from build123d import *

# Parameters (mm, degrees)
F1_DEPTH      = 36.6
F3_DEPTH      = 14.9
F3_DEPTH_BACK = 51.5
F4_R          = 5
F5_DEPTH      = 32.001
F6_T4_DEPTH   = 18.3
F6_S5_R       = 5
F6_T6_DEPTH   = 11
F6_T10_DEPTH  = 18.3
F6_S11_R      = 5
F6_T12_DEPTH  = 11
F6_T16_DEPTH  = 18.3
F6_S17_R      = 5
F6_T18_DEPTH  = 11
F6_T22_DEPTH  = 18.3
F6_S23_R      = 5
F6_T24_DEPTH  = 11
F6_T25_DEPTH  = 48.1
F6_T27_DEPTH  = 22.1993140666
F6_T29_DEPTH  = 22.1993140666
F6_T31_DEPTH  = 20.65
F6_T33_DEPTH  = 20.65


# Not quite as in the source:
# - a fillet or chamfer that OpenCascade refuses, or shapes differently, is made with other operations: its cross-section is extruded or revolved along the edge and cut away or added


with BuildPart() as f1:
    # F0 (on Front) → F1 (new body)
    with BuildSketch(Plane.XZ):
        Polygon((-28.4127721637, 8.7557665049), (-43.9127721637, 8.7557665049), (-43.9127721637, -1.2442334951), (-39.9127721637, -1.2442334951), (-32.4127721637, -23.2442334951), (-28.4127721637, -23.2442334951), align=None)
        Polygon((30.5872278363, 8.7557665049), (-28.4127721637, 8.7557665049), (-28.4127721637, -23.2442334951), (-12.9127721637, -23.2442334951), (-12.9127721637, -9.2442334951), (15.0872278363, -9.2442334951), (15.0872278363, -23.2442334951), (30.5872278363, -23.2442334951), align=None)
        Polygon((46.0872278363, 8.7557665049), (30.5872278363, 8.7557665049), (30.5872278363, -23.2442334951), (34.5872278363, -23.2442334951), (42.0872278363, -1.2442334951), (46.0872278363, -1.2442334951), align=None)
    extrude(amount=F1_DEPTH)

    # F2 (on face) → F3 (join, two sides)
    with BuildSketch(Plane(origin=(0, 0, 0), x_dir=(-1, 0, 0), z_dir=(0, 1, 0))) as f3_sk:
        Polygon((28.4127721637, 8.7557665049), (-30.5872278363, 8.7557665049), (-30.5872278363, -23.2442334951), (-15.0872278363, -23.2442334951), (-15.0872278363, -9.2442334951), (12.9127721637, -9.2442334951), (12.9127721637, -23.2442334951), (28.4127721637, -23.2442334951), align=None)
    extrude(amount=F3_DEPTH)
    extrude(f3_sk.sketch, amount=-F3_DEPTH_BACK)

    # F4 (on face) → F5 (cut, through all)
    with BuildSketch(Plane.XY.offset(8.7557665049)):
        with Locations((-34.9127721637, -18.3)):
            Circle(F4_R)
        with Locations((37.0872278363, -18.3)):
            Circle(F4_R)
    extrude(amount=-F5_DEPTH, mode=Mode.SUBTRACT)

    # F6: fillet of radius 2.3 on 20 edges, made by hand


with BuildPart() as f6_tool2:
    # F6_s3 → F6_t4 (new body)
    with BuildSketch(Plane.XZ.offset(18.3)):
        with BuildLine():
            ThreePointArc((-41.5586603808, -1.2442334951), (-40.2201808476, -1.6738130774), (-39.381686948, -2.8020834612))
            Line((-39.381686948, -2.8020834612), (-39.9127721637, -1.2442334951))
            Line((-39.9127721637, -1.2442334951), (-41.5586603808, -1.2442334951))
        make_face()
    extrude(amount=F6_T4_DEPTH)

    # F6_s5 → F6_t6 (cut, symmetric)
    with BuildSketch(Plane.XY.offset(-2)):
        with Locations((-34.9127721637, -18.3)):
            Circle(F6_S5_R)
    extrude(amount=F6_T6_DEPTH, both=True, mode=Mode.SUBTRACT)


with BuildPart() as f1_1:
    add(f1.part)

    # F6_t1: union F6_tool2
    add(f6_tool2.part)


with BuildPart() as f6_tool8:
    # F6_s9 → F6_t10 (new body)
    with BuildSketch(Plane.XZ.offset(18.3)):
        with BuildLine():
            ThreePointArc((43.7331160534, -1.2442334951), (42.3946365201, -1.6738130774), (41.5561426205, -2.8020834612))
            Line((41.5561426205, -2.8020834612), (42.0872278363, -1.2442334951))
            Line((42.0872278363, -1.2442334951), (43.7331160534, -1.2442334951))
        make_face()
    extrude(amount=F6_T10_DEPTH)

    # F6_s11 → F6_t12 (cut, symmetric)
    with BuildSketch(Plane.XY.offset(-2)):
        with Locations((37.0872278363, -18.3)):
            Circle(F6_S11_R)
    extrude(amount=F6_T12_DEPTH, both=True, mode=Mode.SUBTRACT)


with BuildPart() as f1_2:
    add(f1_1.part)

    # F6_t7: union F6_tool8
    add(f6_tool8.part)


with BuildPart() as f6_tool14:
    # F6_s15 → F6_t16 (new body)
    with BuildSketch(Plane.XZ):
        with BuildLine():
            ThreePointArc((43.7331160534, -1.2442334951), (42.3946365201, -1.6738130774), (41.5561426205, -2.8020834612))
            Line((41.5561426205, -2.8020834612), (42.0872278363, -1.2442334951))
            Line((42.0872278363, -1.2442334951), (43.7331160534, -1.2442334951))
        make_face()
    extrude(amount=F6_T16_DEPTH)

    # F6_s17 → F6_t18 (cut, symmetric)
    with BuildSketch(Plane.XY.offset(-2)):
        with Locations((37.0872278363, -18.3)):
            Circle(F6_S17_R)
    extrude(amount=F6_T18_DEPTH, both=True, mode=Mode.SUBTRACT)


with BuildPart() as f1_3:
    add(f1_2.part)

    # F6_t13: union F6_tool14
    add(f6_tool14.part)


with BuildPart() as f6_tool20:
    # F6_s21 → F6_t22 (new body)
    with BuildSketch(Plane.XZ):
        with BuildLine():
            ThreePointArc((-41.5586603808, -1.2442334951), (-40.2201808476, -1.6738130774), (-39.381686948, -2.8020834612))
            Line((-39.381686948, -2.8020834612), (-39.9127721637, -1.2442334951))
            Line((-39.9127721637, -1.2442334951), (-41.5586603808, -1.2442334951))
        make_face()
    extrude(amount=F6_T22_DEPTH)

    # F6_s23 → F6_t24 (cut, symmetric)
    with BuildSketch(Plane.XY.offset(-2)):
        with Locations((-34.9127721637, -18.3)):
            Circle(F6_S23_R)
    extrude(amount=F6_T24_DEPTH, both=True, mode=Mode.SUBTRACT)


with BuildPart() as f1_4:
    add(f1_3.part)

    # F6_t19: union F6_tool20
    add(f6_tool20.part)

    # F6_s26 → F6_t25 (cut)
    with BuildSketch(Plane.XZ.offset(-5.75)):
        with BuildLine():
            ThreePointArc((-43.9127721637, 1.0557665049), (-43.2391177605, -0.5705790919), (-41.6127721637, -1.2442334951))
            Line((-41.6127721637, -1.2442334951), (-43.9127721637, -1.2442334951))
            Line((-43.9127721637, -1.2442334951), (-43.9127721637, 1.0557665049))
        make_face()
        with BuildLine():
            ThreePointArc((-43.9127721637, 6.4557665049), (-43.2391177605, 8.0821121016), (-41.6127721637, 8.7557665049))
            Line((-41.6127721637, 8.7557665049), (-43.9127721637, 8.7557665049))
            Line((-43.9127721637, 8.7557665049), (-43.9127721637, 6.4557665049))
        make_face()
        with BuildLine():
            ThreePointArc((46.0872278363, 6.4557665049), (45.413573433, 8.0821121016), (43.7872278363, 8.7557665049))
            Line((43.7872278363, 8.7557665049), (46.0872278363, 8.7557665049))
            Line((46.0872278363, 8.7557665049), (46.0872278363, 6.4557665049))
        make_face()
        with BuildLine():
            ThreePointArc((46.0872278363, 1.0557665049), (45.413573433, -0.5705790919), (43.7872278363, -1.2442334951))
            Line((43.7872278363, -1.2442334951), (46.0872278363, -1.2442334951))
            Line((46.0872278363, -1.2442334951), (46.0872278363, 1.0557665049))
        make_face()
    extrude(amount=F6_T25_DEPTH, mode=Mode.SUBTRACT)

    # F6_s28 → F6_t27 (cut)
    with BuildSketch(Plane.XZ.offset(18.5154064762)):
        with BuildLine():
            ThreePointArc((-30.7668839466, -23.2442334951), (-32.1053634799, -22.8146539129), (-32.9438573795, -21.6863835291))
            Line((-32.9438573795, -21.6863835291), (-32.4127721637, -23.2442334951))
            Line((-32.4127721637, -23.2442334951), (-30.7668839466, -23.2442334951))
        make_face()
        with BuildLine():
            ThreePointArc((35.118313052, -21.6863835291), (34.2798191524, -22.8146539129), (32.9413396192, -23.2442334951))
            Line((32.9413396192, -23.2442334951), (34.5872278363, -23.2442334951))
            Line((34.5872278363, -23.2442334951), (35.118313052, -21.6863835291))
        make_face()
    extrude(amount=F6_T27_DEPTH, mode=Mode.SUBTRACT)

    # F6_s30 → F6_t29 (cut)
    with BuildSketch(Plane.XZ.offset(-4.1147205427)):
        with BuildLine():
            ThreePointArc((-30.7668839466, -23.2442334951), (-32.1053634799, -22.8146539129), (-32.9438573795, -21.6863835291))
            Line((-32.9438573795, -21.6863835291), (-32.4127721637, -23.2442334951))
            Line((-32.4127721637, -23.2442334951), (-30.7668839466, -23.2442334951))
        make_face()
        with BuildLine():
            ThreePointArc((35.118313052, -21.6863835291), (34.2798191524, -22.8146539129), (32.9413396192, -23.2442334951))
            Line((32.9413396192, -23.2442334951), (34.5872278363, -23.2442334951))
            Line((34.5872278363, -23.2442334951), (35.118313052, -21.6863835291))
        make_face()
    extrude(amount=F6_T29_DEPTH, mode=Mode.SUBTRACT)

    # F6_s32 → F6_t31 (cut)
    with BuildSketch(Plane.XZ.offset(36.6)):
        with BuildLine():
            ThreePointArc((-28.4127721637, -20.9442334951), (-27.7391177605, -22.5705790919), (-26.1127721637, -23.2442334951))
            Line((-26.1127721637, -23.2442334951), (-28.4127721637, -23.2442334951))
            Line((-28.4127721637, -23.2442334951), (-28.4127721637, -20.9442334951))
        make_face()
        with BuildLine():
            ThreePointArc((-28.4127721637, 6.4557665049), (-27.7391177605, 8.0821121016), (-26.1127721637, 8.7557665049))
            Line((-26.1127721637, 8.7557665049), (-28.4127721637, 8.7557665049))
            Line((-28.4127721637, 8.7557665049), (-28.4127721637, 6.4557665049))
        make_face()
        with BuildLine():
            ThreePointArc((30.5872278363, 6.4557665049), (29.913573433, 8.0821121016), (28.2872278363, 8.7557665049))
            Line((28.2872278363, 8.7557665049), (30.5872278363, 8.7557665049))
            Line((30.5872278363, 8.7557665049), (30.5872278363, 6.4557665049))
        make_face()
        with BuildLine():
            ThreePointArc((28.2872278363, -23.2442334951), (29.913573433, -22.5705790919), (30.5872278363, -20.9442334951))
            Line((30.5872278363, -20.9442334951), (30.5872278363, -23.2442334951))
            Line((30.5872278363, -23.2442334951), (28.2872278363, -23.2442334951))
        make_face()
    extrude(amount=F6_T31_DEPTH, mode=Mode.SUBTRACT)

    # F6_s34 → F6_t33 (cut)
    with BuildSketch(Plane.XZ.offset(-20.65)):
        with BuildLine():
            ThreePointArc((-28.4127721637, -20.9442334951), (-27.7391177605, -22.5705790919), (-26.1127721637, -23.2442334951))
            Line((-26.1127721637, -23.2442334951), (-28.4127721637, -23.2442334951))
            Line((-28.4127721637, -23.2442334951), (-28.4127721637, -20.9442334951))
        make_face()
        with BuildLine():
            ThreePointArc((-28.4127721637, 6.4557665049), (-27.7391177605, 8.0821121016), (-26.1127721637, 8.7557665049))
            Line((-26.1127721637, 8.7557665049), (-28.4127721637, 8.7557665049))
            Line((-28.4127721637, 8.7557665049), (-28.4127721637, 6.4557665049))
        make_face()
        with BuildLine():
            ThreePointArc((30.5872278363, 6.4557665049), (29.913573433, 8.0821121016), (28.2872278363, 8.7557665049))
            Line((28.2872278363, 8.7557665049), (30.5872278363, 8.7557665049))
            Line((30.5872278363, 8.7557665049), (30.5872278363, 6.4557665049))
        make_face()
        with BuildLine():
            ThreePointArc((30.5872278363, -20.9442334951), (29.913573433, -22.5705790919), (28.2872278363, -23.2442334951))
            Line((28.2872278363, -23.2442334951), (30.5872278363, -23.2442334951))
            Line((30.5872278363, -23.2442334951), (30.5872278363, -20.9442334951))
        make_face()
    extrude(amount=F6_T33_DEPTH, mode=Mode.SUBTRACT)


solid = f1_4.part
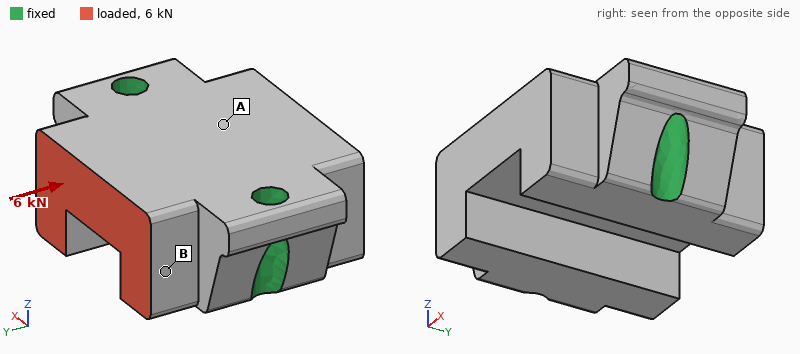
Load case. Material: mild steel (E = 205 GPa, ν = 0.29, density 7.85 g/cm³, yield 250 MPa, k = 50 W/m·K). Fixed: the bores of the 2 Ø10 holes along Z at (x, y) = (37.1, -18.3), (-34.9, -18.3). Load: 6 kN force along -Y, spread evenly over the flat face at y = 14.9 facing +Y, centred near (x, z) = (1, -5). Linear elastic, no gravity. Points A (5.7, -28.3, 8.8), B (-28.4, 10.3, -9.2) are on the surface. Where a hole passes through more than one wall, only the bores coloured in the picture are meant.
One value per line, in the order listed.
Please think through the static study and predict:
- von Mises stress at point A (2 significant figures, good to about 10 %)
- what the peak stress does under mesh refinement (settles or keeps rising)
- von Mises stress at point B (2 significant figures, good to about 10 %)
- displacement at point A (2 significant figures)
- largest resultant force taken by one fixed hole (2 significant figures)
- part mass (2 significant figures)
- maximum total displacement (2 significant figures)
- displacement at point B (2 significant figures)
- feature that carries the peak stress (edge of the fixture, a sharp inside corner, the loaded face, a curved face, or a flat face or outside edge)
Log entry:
2.0 MPa
keeps rising
4.7 MPa
0.83 µm
3.0 kN
930 g
1.5 µm
0.82 µm
edge of the fixture
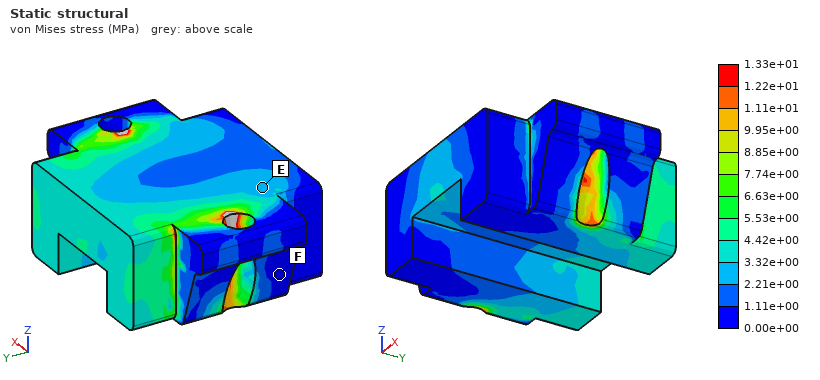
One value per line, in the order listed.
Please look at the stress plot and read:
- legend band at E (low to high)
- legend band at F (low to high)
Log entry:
2.21e+00 to 3.32e+00 MPa
0.00e+00 to 1.11e+00 MPa
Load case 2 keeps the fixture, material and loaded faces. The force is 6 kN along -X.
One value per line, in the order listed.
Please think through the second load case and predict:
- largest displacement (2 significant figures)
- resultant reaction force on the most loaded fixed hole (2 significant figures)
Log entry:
4.1 µm
4.0 kN
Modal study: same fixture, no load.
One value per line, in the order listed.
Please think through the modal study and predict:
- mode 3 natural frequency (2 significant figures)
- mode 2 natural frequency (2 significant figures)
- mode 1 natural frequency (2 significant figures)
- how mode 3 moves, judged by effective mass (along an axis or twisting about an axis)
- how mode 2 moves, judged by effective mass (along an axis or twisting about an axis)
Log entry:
16 kHz
13 kHz
11 kHz
along Y
along Z
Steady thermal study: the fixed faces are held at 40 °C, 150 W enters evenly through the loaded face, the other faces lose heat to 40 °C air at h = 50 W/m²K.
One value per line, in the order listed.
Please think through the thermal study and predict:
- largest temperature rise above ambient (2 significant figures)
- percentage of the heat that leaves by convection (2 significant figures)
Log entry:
70 K
11 %
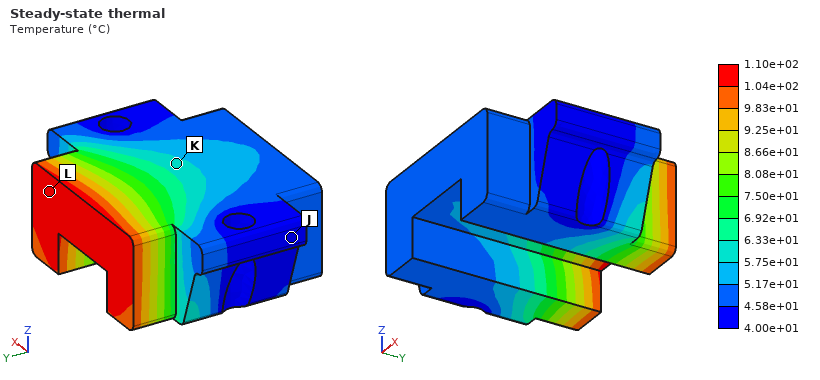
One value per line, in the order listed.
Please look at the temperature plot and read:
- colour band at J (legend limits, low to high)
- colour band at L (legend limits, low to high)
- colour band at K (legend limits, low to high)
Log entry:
4.00e+01 to 4.58e+01 °C
1.04e+02 to 1.10e+02 °C
5.75e+01 to 6.33e+01 °C
